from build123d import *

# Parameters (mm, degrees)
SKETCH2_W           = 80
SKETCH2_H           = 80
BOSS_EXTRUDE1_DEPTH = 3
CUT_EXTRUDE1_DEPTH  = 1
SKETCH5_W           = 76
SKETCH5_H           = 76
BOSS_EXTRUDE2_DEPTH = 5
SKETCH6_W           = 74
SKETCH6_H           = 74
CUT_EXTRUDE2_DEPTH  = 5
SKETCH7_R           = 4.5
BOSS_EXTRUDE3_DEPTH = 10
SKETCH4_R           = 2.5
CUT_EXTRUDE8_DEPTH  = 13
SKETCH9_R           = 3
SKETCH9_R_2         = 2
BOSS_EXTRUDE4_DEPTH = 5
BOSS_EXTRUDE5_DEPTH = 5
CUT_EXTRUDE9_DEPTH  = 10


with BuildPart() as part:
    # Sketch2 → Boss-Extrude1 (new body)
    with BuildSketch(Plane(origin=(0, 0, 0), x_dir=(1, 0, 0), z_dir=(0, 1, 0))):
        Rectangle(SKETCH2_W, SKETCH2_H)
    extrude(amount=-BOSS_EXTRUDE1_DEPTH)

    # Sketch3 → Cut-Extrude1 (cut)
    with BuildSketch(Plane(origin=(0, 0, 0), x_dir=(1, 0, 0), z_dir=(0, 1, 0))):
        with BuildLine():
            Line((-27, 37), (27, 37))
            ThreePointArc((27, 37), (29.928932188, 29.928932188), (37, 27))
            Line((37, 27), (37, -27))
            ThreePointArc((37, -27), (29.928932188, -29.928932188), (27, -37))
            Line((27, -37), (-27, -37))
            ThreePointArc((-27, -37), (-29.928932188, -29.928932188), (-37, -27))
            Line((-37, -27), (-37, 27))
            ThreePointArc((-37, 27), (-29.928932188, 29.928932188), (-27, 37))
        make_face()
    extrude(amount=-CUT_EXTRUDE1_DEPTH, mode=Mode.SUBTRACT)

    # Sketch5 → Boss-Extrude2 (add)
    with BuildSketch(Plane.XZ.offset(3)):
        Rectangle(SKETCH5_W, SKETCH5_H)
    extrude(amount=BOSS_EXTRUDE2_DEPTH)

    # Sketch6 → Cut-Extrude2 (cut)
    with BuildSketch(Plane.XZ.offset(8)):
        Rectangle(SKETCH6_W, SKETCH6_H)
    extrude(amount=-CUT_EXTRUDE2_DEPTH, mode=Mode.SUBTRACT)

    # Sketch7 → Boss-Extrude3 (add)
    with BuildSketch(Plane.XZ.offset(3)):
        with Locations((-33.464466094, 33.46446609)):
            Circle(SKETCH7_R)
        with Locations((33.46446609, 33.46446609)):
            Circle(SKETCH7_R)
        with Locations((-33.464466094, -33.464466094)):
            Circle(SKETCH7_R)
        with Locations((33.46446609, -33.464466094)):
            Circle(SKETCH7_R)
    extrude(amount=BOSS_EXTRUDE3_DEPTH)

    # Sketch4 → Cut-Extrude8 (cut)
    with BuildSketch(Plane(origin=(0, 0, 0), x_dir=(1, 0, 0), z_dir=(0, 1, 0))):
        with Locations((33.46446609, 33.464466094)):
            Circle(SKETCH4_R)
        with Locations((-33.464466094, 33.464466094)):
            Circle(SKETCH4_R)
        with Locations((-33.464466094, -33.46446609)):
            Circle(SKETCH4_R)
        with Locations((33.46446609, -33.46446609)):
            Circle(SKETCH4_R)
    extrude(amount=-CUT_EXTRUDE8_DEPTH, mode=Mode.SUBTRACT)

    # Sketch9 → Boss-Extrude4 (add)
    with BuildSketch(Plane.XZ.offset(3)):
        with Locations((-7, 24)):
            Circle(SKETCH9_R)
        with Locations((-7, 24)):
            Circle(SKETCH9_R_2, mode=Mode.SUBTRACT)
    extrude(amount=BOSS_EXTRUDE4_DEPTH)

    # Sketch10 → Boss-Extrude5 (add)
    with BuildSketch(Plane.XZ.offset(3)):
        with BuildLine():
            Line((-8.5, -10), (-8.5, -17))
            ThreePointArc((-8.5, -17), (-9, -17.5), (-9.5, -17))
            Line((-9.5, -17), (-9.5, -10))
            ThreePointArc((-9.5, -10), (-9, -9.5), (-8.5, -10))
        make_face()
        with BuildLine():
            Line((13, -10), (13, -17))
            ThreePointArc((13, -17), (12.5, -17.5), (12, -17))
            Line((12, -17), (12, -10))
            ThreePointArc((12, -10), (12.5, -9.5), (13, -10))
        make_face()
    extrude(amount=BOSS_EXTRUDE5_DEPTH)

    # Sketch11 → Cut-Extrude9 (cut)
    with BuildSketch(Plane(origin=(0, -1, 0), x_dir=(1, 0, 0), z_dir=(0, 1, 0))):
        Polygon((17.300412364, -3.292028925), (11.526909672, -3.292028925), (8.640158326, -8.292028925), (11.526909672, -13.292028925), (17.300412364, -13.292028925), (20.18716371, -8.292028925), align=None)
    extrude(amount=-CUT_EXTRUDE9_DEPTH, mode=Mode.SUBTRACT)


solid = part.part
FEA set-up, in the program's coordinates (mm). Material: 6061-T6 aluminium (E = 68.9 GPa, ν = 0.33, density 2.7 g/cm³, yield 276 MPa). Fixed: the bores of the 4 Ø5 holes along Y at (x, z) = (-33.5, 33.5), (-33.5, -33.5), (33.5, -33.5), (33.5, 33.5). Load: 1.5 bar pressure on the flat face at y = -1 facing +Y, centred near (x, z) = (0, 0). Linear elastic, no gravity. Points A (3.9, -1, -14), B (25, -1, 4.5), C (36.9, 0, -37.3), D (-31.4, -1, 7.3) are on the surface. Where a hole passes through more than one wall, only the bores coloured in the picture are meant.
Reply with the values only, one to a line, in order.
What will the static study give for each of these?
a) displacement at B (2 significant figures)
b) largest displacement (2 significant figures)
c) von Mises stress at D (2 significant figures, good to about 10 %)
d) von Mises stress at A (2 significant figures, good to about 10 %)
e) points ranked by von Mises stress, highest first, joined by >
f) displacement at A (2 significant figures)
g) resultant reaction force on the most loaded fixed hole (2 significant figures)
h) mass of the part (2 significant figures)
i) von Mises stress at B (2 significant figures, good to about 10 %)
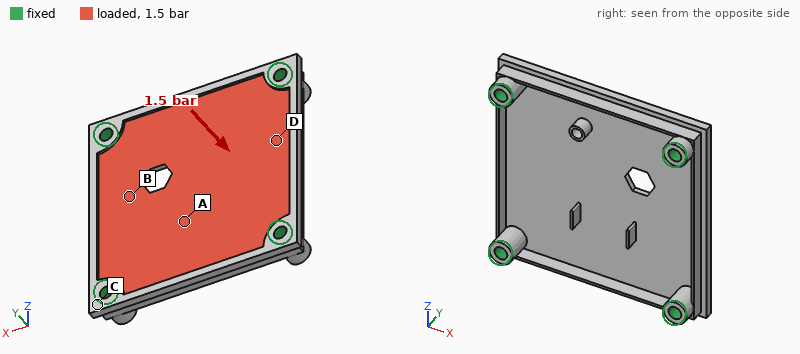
0.13 mm
0.24 mm
18 MPa
35 MPa
A > B > D > C
0.19 mm
190 N
46 g
25 MPa
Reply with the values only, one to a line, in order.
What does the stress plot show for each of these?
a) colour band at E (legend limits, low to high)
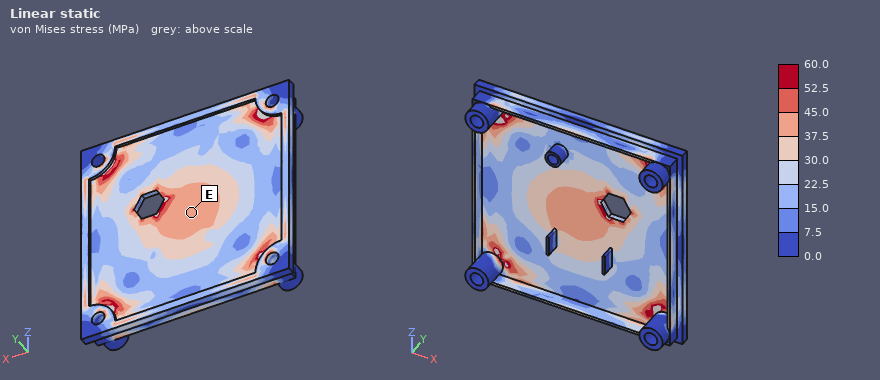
37.5 to 45.0 MPa
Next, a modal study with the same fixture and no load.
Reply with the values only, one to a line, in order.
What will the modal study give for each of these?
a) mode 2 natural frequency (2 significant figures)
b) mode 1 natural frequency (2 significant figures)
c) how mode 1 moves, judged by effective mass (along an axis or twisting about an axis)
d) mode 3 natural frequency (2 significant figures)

4500 Hz
2100 Hz
along Y
4500 Hz
